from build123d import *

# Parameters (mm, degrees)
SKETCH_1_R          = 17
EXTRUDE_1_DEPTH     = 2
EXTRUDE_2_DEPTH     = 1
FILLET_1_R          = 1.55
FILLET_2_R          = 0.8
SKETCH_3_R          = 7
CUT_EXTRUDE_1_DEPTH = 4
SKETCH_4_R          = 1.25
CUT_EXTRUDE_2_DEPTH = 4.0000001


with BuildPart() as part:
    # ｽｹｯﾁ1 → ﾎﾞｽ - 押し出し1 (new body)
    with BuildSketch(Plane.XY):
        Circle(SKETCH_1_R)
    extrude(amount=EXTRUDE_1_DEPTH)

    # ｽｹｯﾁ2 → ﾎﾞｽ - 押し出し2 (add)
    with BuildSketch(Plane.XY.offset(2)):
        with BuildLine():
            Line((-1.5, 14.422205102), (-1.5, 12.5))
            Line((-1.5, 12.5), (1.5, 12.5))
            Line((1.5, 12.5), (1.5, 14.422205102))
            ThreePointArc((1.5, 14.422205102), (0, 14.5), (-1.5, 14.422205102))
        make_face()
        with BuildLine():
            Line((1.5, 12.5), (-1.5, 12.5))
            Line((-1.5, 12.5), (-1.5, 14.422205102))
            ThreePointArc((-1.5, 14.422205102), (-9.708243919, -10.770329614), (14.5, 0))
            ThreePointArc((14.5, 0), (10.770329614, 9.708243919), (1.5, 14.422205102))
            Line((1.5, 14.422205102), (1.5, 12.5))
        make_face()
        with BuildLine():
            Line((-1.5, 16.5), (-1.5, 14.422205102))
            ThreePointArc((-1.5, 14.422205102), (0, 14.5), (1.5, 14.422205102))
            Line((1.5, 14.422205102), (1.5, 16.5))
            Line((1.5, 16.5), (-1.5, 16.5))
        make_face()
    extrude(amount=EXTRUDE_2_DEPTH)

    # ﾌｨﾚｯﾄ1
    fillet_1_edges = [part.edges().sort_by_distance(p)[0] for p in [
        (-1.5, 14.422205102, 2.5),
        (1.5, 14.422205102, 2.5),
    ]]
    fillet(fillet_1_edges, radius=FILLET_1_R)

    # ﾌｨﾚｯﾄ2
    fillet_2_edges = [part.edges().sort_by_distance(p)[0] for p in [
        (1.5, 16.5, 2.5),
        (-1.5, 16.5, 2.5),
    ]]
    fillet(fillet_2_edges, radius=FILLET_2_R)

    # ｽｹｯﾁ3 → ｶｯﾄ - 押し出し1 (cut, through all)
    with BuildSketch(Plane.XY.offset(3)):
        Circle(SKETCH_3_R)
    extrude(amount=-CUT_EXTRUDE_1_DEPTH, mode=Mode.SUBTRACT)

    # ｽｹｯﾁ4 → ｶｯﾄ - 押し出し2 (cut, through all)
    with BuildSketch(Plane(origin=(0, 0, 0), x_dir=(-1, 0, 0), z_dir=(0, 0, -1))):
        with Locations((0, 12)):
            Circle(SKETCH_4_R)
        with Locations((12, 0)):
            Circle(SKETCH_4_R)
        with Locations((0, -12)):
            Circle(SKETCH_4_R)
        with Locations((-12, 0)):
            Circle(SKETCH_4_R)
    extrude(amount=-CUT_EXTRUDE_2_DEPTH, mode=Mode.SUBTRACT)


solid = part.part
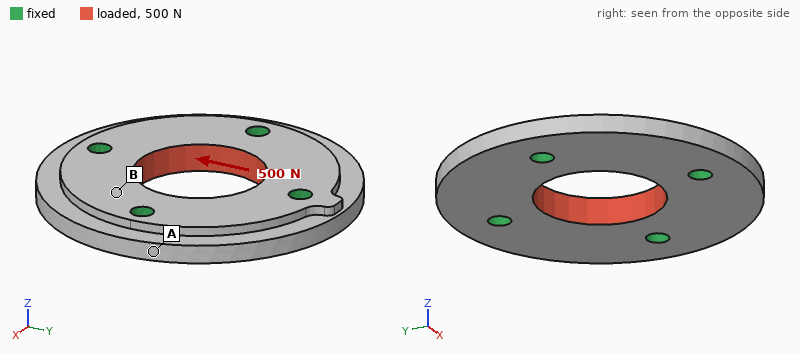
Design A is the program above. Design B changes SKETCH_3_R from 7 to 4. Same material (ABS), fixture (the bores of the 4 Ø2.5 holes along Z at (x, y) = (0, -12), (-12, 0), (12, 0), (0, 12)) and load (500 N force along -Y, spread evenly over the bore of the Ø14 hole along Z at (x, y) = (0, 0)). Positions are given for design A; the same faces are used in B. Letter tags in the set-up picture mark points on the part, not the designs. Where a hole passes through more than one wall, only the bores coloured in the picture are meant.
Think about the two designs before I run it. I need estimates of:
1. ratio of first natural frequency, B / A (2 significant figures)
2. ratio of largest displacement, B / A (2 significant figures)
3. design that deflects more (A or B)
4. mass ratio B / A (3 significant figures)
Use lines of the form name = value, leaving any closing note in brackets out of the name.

ratio of first natural frequency, B / A = 1.0
ratio of largest displacement, B / A = 1.4
design that deflects more = B
mass ratio B / A = 1.16
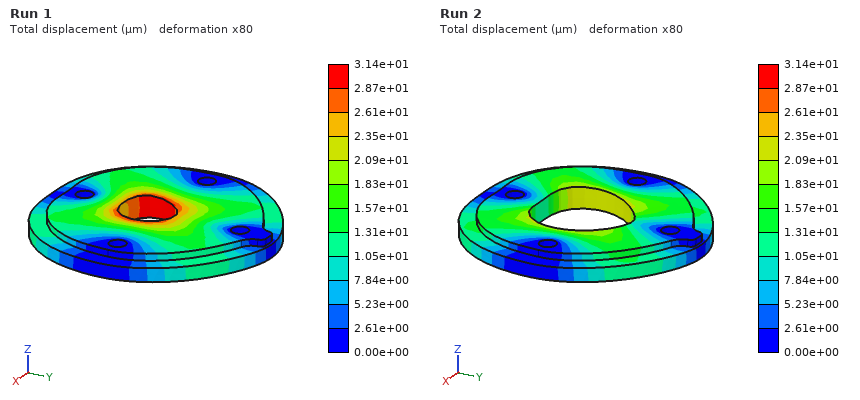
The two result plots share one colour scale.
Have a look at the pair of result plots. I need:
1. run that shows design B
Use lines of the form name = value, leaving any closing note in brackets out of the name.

run that shows design B = Run 1
